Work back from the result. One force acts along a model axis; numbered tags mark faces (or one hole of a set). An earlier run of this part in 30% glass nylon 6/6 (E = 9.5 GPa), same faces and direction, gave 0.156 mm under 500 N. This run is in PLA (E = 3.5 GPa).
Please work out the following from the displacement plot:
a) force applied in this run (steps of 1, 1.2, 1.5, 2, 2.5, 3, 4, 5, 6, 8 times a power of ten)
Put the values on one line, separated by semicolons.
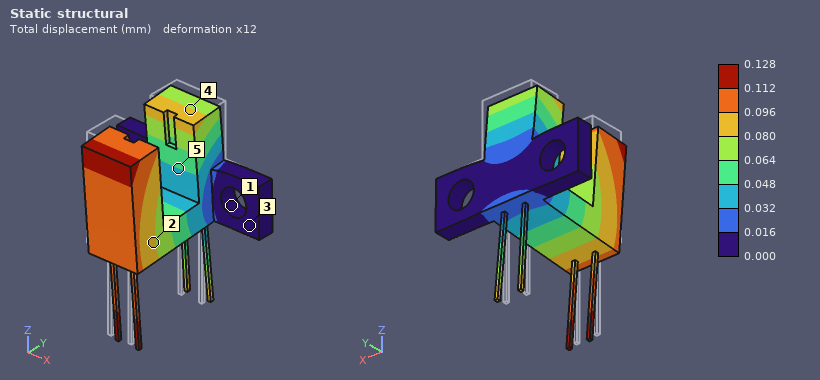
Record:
150 N
